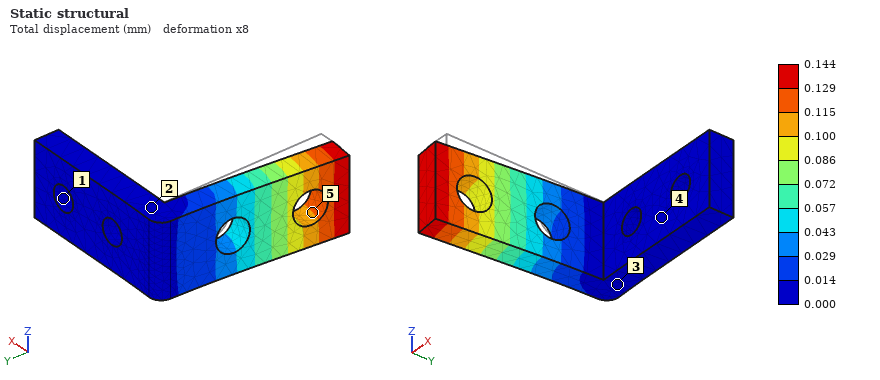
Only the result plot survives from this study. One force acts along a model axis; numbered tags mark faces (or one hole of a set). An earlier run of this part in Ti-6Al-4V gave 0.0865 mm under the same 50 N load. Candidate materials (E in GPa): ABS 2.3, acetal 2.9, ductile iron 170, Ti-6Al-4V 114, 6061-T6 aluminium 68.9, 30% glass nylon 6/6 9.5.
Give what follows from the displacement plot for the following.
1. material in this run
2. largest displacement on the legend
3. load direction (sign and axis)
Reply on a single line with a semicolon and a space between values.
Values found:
6061-T6 aluminium; 0.144 mm; -X
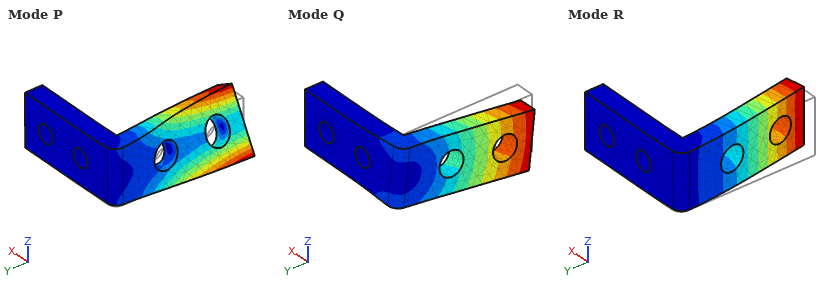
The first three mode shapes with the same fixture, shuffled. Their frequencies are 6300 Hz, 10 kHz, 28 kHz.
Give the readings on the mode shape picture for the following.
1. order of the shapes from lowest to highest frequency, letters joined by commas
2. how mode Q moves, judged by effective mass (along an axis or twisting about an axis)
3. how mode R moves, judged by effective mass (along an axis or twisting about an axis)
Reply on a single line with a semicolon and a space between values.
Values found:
R, Q, P; along Z; along X
